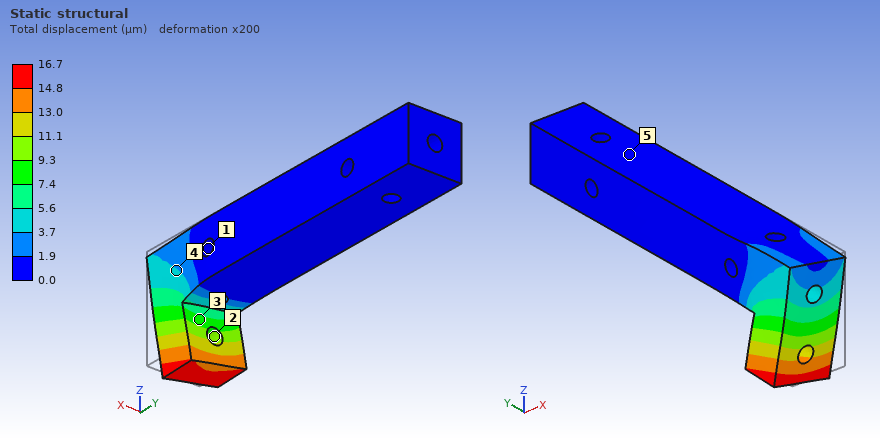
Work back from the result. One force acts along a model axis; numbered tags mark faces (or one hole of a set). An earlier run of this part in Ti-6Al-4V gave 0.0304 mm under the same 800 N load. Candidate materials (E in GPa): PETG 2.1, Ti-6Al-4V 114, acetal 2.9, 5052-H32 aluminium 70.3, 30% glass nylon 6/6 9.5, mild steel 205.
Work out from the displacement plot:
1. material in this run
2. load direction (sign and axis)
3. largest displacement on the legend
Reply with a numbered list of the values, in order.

1. mild steel
2. -X
3. 16.7 µm
